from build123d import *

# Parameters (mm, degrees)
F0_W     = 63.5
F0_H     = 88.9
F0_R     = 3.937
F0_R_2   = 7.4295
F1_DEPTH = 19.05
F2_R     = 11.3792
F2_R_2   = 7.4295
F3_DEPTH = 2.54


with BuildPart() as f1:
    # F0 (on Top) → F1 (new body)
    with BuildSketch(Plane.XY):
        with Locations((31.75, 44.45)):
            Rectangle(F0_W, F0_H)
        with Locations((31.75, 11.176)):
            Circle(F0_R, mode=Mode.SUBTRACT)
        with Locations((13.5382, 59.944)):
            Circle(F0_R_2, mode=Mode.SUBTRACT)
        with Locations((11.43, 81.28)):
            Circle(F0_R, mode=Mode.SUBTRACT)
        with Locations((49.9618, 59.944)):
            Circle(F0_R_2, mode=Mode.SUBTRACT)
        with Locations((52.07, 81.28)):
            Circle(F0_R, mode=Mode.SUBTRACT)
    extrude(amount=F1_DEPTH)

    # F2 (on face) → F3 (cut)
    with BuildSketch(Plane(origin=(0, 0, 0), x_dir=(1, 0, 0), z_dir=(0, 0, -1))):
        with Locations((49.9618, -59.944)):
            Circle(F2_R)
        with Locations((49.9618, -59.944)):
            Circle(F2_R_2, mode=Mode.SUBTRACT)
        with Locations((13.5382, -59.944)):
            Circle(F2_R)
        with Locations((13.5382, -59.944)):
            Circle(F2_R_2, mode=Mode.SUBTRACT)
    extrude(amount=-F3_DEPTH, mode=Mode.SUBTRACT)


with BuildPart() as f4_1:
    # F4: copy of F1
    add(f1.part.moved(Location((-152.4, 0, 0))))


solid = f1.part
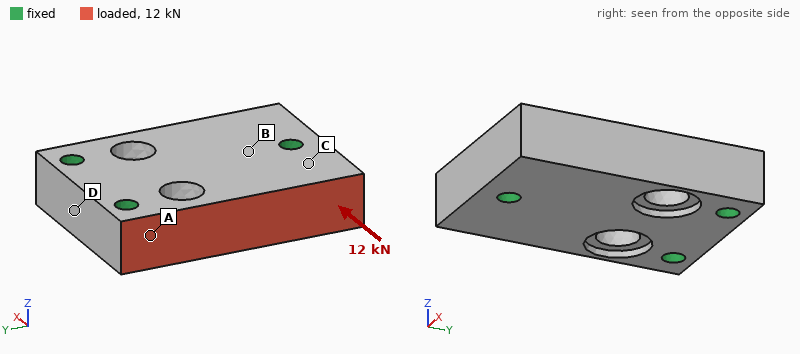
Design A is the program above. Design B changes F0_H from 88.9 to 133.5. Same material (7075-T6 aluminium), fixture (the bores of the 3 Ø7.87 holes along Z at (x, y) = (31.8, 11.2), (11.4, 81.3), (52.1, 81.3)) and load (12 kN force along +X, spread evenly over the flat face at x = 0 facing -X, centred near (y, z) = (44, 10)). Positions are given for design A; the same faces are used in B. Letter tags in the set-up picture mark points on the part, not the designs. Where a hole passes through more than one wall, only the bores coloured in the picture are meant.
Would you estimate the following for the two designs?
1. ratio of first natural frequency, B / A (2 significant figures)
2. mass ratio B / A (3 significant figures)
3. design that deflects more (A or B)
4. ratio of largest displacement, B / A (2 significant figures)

0.81
1.56
A
0.65
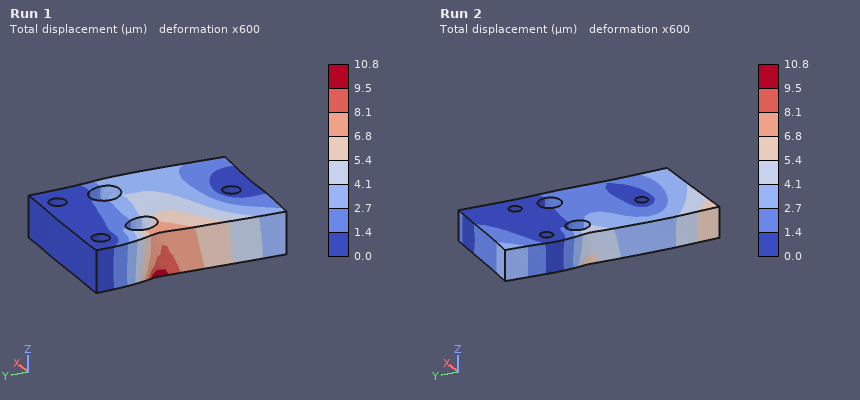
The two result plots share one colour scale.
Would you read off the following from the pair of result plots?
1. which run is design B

Run 2
